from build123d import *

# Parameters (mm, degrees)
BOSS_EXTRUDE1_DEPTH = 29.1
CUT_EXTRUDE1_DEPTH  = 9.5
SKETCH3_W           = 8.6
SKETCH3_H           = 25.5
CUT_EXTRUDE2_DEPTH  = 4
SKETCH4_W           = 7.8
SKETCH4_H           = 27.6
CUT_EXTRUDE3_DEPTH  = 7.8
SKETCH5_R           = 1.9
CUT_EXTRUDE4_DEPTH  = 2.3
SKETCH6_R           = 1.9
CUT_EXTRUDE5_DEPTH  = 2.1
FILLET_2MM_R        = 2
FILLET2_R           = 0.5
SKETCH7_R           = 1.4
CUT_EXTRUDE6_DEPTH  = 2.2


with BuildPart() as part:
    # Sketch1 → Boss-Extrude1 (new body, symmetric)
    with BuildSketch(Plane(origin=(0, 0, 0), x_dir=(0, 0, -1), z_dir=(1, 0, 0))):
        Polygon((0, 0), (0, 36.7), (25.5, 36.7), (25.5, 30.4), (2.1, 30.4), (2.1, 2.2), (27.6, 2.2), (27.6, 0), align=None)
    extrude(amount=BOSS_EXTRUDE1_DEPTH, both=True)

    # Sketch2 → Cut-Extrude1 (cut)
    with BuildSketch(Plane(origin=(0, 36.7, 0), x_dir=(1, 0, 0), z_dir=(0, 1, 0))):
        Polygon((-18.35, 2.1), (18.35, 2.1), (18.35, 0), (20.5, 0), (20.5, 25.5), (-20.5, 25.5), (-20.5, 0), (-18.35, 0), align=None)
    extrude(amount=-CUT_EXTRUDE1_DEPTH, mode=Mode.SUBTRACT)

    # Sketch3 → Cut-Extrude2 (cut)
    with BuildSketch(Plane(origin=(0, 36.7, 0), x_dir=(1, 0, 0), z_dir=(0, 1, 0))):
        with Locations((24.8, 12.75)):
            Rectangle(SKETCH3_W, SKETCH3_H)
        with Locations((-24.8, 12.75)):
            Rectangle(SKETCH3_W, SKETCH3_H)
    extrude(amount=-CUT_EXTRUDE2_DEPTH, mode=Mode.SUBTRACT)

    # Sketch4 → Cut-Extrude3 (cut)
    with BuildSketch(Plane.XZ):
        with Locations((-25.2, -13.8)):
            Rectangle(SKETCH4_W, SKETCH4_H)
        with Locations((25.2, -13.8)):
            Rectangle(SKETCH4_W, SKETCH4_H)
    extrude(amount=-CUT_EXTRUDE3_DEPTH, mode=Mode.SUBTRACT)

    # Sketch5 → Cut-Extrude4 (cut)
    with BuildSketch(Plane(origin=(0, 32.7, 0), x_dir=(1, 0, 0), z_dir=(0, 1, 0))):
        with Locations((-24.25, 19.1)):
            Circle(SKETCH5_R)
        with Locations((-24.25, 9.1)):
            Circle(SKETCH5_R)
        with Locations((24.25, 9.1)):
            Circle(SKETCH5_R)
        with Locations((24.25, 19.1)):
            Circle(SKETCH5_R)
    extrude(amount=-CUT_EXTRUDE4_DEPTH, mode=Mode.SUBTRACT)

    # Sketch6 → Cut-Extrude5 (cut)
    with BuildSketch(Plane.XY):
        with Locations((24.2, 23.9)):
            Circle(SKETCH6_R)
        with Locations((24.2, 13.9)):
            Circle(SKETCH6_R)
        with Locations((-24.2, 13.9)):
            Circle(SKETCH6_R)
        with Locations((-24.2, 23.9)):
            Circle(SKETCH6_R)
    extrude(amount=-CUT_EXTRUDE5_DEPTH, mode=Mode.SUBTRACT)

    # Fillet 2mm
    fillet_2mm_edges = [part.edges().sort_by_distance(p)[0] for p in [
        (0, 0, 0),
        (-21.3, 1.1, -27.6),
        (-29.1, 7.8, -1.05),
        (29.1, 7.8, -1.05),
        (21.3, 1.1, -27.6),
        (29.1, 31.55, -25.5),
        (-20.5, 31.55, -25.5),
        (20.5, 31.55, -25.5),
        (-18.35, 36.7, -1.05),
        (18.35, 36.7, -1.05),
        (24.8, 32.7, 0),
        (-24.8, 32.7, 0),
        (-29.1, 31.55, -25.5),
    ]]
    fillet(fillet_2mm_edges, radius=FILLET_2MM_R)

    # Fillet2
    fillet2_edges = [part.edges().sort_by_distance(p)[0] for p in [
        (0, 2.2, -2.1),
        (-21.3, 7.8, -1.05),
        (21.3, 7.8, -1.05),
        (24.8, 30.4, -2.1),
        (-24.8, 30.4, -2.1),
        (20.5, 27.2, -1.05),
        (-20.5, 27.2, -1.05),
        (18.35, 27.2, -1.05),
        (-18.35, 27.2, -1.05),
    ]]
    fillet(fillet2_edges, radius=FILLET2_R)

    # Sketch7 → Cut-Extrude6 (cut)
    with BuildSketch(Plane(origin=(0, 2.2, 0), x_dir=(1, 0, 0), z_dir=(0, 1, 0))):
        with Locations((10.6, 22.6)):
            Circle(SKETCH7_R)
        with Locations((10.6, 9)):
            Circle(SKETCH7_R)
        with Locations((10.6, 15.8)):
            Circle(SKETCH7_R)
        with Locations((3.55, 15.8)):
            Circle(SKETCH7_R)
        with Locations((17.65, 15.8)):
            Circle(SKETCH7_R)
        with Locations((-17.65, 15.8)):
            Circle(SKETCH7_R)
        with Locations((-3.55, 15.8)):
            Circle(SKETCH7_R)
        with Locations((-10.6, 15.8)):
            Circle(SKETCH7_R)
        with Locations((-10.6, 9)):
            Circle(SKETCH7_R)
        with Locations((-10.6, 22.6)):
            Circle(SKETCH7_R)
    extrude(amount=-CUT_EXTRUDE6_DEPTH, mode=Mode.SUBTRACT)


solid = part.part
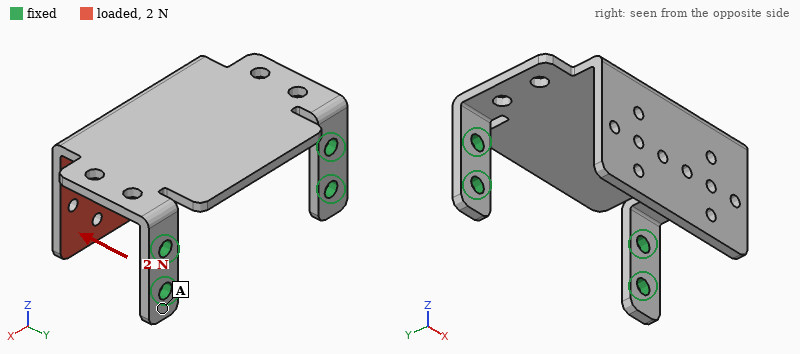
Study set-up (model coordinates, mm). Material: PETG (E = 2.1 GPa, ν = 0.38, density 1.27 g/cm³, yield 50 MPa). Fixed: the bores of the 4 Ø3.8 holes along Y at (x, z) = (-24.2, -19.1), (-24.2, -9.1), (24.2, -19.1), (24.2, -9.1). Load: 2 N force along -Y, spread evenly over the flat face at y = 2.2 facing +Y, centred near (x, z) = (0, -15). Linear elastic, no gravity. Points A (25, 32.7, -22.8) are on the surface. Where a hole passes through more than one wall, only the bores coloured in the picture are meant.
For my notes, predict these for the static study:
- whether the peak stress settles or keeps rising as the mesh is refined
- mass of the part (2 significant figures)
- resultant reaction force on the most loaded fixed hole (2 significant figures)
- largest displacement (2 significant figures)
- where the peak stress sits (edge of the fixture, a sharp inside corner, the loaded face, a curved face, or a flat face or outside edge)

keeps rising
8.8 g
1.0 N
0.75 mm
a sharp inside corner
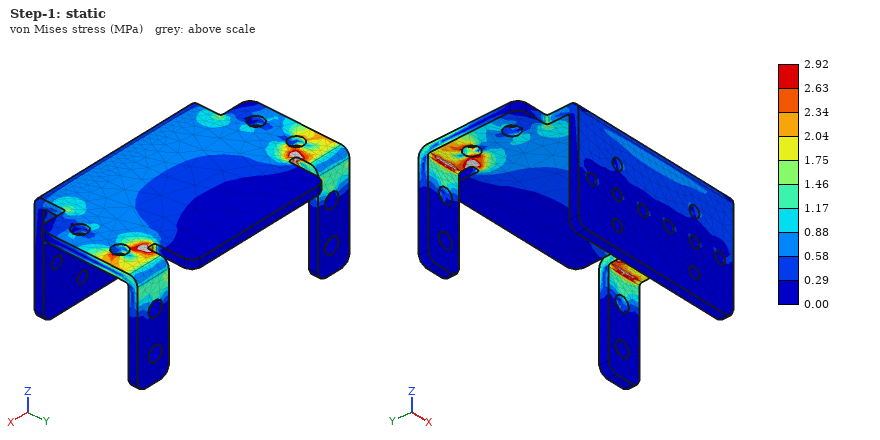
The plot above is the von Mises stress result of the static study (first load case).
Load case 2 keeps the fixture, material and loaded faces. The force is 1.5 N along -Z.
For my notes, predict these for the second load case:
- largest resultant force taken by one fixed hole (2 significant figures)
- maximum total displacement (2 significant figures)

0.74 N
0.89 mm
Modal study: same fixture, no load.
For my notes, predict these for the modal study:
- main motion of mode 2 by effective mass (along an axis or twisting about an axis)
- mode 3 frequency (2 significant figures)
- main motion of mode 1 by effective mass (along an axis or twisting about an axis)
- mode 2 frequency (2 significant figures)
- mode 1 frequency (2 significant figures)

along X
420 Hz
along Z
320 Hz
110 Hz
